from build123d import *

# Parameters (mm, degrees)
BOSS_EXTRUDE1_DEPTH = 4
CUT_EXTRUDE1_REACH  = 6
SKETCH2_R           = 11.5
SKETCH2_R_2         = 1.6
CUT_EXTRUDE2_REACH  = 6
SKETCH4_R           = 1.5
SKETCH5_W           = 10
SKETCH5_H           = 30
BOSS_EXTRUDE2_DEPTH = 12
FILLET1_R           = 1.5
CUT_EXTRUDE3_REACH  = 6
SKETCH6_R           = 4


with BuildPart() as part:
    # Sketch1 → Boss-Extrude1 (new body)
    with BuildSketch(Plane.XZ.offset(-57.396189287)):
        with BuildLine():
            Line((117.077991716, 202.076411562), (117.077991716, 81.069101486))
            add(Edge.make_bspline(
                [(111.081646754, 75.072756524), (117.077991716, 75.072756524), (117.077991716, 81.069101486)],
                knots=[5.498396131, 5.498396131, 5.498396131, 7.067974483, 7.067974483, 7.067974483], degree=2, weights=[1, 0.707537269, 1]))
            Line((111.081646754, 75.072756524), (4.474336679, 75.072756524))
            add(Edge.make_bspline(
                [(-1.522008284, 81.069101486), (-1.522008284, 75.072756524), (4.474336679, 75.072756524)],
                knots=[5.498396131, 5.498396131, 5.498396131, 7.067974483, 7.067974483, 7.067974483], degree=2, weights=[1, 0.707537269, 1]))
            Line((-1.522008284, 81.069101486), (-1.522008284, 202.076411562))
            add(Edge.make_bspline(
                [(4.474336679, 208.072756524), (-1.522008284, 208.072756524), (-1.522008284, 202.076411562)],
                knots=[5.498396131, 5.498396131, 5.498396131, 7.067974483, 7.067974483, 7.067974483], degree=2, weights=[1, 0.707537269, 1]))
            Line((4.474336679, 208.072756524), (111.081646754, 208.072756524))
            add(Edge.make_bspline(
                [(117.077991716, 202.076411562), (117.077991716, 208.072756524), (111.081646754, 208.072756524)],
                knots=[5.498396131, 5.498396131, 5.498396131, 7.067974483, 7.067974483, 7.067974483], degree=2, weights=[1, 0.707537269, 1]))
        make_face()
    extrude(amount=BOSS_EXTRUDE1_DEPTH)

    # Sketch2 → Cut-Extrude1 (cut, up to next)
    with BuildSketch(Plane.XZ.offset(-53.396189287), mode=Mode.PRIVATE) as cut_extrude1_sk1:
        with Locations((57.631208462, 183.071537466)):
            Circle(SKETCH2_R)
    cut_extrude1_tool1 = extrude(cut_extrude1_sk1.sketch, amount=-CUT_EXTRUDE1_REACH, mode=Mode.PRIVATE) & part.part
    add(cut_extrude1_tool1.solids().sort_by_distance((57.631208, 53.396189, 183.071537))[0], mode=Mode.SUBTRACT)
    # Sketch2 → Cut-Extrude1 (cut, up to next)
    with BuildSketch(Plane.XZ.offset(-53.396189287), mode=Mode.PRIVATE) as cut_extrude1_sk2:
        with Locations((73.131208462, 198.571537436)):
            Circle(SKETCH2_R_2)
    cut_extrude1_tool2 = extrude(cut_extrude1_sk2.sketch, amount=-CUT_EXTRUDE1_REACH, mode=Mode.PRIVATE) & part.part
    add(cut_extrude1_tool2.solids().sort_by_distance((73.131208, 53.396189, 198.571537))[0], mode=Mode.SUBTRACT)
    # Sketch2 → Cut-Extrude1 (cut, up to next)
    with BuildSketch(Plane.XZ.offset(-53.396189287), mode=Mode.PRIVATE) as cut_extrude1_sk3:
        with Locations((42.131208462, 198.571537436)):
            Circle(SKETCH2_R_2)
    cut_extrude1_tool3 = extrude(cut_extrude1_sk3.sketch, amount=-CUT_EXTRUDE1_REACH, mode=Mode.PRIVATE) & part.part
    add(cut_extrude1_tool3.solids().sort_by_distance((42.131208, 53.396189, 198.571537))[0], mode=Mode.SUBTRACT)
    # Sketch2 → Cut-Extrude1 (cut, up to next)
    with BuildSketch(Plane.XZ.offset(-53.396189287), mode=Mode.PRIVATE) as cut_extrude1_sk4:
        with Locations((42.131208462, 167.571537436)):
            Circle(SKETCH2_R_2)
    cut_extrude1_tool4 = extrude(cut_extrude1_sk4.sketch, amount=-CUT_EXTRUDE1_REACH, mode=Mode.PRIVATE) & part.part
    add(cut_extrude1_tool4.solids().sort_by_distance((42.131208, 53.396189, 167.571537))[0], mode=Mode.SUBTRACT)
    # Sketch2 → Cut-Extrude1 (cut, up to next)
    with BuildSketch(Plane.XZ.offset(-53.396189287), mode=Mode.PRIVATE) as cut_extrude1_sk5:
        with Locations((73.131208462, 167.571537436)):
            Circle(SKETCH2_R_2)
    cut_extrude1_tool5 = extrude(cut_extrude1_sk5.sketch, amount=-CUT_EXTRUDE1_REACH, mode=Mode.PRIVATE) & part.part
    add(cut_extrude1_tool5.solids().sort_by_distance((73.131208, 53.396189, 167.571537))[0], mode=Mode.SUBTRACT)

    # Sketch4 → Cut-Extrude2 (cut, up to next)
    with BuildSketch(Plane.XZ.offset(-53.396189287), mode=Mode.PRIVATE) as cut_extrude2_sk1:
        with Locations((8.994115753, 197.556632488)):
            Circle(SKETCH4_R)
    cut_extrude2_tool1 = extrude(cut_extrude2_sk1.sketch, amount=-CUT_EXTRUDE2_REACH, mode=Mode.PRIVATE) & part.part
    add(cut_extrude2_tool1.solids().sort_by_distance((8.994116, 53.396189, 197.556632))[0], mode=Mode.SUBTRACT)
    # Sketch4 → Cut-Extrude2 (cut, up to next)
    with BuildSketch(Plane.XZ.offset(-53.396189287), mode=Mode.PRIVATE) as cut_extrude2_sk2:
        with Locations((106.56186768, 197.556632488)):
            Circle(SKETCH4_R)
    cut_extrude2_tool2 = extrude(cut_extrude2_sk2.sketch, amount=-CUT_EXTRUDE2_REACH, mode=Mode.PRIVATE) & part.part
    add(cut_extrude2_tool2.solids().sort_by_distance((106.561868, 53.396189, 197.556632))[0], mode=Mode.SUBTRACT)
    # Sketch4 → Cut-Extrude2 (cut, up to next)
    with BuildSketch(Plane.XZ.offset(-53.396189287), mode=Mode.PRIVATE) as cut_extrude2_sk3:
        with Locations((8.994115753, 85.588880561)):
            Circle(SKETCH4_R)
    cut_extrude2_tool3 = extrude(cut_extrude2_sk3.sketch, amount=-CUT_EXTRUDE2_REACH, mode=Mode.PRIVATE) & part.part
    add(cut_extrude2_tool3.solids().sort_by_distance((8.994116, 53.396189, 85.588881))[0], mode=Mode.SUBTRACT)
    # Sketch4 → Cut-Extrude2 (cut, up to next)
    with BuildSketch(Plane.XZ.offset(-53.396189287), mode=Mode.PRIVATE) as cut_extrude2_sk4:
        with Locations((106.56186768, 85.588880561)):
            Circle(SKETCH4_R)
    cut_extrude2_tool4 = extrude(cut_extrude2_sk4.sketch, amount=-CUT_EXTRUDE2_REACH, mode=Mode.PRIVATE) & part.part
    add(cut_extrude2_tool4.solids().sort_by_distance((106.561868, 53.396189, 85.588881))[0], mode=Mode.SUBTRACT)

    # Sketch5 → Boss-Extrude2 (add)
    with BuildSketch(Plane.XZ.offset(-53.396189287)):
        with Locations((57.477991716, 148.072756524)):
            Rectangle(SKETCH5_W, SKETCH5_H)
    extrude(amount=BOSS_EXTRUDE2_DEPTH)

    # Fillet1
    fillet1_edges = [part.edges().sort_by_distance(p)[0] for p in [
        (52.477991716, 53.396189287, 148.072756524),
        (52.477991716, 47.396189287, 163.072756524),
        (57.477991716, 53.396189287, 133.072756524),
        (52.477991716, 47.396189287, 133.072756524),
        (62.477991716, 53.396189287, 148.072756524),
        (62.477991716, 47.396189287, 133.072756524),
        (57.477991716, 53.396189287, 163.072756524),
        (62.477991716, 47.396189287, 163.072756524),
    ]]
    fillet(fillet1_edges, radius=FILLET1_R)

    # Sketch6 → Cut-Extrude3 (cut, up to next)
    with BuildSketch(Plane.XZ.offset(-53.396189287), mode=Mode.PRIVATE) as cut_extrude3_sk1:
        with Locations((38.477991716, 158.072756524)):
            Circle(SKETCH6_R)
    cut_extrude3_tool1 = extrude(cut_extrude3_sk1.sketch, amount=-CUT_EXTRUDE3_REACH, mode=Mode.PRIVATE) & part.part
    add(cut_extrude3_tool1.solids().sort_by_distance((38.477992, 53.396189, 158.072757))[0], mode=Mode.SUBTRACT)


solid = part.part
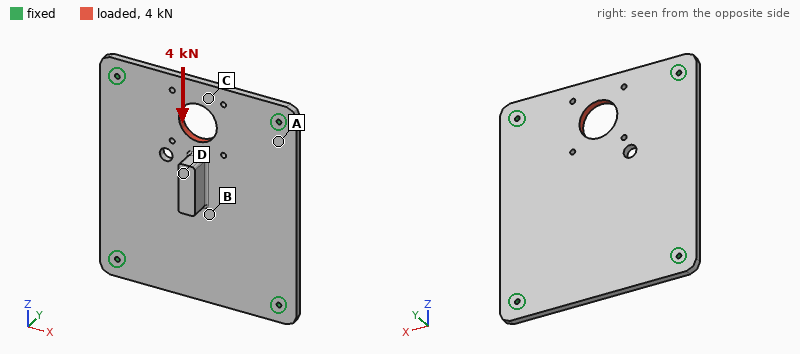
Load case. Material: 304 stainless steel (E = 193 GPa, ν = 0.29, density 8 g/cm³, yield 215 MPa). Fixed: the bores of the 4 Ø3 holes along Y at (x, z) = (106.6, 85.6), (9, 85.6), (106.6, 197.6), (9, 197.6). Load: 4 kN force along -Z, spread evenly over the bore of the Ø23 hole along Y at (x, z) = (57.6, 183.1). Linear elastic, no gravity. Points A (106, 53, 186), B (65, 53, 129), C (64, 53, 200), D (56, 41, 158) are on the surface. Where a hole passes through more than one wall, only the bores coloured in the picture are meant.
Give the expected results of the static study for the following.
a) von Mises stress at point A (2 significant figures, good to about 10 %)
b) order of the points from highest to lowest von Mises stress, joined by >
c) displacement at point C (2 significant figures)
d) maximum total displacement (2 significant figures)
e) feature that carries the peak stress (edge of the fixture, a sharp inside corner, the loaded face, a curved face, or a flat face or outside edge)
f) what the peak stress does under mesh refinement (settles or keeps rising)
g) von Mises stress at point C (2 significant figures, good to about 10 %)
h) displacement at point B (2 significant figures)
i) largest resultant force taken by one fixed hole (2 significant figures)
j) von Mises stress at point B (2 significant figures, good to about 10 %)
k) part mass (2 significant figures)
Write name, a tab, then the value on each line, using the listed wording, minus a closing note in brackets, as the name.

von Mises stress at point A	12 MPa
order of the points from highest to lowest von Mises stress, joined by >	C > A > B > D
displacement at point C	7.7 µm
maximum total displacement	8.6 µm
feature that carries the peak stress	edge of the fixture
what the peak stress does under mesh refinement	keeps rising
von Mises stress at point C	17 MPa
displacement at point B	2.8 µm
largest resultant force taken by one fixed hole	1.2 kN
von Mises stress at point B	6.9 MPa
part mass	520 g
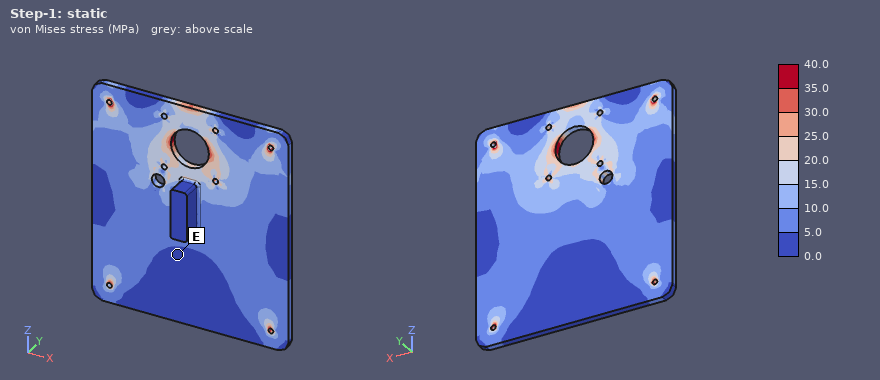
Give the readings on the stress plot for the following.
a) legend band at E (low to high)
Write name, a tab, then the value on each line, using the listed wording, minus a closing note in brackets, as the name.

legend band at E	0.0 to 5.0 MPa
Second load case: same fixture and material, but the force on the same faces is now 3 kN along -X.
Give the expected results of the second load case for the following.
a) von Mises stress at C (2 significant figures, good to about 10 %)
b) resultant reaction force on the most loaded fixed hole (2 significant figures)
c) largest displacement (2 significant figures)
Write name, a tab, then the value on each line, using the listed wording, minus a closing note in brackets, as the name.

von Mises stress at C	8.1 MPa
resultant reaction force on the most loaded fixed hole	1.2 kN
largest displacement	3.5 µm
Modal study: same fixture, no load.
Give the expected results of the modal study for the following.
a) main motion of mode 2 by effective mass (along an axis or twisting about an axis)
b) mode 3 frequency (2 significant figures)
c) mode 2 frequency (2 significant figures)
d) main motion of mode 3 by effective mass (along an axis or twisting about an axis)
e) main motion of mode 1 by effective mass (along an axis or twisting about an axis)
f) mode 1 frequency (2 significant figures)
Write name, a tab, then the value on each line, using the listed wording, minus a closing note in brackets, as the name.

main motion of mode 2 by effective mass	twisting about Z
mode 3 frequency	2000 Hz
mode 2 frequency	1700 Hz
main motion of mode 3 by effective mass	twisting about X
main motion of mode 1 by effective mass	along Y
mode 1 frequency	1000 Hz
